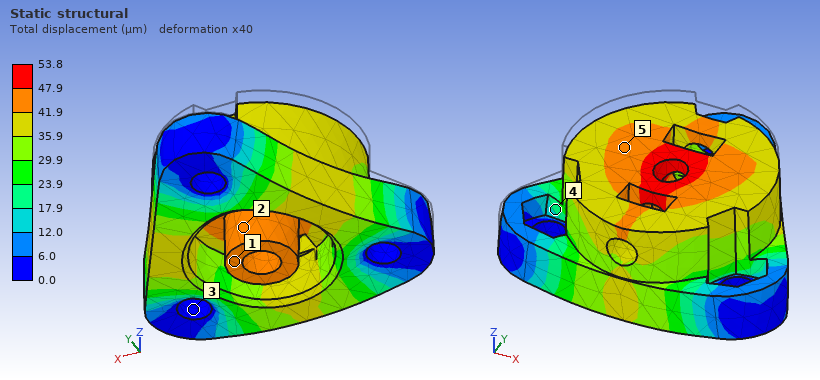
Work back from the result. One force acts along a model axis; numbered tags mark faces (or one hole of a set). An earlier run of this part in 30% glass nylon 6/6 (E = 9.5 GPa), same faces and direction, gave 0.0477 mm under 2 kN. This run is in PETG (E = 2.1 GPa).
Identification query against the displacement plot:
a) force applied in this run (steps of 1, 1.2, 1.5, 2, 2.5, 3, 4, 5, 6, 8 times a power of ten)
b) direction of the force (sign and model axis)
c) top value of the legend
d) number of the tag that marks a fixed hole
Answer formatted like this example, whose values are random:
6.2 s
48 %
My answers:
500 N
-Z
53.8 µm
3
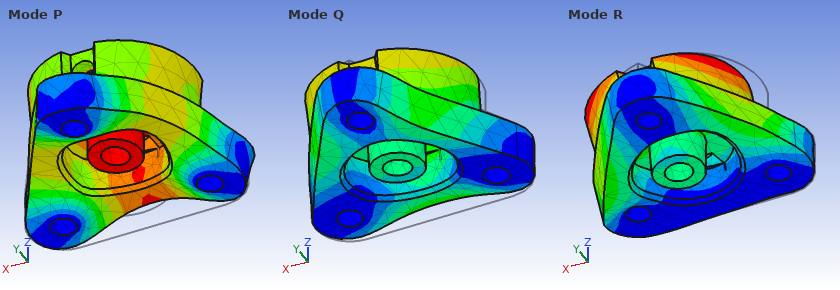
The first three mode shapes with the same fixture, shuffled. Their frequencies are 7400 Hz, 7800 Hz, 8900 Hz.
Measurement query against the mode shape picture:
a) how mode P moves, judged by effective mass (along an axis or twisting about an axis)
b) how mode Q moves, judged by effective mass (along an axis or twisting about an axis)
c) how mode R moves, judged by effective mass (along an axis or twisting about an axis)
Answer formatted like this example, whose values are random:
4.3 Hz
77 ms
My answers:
along Z
along Y
along X
